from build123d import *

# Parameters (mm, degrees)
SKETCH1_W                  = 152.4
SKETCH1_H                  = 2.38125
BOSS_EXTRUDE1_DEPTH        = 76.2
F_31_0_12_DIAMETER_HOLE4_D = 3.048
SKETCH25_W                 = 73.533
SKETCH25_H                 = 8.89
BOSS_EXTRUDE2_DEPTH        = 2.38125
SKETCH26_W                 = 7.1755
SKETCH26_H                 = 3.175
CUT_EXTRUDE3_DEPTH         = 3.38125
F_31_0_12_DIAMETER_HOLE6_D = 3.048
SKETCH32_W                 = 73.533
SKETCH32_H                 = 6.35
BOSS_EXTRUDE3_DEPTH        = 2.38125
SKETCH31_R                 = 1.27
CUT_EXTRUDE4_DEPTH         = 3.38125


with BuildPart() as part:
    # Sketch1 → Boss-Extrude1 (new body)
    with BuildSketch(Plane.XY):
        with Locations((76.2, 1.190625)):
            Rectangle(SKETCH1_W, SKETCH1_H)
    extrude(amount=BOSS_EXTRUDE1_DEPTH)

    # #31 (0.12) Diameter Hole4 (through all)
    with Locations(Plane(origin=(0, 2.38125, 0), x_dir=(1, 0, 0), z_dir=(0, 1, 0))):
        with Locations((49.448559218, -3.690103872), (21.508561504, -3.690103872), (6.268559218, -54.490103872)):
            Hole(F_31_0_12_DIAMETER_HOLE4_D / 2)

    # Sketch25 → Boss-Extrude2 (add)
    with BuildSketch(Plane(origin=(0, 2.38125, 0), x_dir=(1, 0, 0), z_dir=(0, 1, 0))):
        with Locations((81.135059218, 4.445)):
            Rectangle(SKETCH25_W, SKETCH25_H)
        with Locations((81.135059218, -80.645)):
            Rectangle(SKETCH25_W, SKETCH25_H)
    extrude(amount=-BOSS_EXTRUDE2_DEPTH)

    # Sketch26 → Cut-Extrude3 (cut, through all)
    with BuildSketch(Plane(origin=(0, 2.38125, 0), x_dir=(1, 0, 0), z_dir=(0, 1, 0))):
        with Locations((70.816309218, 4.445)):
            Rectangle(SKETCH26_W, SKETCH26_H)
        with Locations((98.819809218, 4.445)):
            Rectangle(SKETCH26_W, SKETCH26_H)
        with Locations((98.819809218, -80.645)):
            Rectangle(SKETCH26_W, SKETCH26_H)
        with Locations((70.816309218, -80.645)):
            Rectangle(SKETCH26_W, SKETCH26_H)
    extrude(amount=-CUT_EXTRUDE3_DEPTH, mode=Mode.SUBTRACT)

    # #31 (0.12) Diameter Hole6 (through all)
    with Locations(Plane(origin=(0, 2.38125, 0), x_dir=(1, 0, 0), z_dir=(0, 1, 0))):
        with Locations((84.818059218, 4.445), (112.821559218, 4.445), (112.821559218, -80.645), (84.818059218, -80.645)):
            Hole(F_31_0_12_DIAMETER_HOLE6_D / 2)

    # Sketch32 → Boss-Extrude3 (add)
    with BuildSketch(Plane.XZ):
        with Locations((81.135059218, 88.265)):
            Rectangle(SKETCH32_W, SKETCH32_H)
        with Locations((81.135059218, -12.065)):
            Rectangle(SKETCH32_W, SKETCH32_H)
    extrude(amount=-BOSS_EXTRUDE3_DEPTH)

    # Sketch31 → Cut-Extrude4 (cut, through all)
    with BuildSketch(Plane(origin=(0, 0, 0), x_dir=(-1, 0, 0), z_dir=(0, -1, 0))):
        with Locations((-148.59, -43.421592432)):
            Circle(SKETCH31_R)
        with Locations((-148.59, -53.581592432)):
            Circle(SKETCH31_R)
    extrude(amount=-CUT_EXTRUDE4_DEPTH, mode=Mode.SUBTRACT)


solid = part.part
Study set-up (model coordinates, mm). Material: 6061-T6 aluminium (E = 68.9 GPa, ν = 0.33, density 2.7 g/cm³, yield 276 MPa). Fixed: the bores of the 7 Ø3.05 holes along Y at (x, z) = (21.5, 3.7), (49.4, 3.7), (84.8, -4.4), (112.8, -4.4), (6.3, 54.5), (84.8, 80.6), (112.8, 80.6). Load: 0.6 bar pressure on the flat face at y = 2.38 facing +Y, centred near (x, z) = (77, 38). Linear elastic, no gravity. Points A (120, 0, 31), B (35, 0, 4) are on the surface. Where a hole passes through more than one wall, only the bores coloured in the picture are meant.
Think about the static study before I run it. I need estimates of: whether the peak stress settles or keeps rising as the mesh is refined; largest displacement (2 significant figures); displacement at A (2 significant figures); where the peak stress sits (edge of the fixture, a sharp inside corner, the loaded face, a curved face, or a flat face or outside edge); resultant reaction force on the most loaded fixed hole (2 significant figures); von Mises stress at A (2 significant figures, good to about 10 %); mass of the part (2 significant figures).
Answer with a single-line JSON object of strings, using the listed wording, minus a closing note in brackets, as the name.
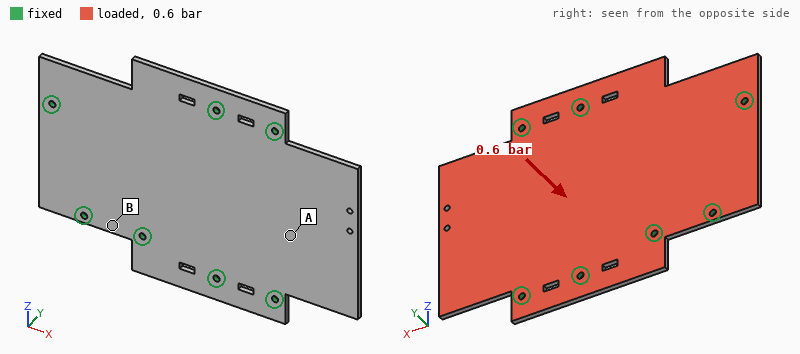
{"whether the peak stress settles or keeps rising as the mesh is refined": "keeps rising", "largest displacement": "0.68 mm", "displacement at A": "0.26 mm", "where the peak stress sits": "edge of the fixture", "resultant reaction force on the most loaded fixed hole": "170 N", "von Mises stress at A": "35 MPa", "mass of the part": "88 g"}
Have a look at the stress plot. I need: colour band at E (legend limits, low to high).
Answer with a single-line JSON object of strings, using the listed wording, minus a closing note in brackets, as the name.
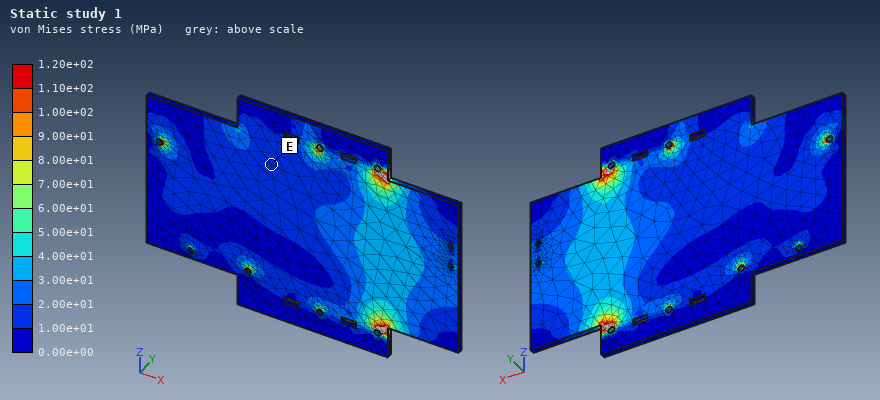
{"colour band at E": "1.00e+01 to 2.00e+01 MPa"}
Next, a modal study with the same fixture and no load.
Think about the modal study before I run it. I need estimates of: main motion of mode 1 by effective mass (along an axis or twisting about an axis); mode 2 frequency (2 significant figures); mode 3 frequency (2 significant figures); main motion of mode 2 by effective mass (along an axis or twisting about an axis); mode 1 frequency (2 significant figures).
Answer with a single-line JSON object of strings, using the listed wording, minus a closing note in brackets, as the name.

{"main motion of mode 1 by effective mass": "along Y", "mode 2 frequency": "1600 Hz", "mode 3 frequency": "1700 Hz", "main motion of mode 2 by effective mass": "along Y", "mode 1 frequency": "760 Hz"}
